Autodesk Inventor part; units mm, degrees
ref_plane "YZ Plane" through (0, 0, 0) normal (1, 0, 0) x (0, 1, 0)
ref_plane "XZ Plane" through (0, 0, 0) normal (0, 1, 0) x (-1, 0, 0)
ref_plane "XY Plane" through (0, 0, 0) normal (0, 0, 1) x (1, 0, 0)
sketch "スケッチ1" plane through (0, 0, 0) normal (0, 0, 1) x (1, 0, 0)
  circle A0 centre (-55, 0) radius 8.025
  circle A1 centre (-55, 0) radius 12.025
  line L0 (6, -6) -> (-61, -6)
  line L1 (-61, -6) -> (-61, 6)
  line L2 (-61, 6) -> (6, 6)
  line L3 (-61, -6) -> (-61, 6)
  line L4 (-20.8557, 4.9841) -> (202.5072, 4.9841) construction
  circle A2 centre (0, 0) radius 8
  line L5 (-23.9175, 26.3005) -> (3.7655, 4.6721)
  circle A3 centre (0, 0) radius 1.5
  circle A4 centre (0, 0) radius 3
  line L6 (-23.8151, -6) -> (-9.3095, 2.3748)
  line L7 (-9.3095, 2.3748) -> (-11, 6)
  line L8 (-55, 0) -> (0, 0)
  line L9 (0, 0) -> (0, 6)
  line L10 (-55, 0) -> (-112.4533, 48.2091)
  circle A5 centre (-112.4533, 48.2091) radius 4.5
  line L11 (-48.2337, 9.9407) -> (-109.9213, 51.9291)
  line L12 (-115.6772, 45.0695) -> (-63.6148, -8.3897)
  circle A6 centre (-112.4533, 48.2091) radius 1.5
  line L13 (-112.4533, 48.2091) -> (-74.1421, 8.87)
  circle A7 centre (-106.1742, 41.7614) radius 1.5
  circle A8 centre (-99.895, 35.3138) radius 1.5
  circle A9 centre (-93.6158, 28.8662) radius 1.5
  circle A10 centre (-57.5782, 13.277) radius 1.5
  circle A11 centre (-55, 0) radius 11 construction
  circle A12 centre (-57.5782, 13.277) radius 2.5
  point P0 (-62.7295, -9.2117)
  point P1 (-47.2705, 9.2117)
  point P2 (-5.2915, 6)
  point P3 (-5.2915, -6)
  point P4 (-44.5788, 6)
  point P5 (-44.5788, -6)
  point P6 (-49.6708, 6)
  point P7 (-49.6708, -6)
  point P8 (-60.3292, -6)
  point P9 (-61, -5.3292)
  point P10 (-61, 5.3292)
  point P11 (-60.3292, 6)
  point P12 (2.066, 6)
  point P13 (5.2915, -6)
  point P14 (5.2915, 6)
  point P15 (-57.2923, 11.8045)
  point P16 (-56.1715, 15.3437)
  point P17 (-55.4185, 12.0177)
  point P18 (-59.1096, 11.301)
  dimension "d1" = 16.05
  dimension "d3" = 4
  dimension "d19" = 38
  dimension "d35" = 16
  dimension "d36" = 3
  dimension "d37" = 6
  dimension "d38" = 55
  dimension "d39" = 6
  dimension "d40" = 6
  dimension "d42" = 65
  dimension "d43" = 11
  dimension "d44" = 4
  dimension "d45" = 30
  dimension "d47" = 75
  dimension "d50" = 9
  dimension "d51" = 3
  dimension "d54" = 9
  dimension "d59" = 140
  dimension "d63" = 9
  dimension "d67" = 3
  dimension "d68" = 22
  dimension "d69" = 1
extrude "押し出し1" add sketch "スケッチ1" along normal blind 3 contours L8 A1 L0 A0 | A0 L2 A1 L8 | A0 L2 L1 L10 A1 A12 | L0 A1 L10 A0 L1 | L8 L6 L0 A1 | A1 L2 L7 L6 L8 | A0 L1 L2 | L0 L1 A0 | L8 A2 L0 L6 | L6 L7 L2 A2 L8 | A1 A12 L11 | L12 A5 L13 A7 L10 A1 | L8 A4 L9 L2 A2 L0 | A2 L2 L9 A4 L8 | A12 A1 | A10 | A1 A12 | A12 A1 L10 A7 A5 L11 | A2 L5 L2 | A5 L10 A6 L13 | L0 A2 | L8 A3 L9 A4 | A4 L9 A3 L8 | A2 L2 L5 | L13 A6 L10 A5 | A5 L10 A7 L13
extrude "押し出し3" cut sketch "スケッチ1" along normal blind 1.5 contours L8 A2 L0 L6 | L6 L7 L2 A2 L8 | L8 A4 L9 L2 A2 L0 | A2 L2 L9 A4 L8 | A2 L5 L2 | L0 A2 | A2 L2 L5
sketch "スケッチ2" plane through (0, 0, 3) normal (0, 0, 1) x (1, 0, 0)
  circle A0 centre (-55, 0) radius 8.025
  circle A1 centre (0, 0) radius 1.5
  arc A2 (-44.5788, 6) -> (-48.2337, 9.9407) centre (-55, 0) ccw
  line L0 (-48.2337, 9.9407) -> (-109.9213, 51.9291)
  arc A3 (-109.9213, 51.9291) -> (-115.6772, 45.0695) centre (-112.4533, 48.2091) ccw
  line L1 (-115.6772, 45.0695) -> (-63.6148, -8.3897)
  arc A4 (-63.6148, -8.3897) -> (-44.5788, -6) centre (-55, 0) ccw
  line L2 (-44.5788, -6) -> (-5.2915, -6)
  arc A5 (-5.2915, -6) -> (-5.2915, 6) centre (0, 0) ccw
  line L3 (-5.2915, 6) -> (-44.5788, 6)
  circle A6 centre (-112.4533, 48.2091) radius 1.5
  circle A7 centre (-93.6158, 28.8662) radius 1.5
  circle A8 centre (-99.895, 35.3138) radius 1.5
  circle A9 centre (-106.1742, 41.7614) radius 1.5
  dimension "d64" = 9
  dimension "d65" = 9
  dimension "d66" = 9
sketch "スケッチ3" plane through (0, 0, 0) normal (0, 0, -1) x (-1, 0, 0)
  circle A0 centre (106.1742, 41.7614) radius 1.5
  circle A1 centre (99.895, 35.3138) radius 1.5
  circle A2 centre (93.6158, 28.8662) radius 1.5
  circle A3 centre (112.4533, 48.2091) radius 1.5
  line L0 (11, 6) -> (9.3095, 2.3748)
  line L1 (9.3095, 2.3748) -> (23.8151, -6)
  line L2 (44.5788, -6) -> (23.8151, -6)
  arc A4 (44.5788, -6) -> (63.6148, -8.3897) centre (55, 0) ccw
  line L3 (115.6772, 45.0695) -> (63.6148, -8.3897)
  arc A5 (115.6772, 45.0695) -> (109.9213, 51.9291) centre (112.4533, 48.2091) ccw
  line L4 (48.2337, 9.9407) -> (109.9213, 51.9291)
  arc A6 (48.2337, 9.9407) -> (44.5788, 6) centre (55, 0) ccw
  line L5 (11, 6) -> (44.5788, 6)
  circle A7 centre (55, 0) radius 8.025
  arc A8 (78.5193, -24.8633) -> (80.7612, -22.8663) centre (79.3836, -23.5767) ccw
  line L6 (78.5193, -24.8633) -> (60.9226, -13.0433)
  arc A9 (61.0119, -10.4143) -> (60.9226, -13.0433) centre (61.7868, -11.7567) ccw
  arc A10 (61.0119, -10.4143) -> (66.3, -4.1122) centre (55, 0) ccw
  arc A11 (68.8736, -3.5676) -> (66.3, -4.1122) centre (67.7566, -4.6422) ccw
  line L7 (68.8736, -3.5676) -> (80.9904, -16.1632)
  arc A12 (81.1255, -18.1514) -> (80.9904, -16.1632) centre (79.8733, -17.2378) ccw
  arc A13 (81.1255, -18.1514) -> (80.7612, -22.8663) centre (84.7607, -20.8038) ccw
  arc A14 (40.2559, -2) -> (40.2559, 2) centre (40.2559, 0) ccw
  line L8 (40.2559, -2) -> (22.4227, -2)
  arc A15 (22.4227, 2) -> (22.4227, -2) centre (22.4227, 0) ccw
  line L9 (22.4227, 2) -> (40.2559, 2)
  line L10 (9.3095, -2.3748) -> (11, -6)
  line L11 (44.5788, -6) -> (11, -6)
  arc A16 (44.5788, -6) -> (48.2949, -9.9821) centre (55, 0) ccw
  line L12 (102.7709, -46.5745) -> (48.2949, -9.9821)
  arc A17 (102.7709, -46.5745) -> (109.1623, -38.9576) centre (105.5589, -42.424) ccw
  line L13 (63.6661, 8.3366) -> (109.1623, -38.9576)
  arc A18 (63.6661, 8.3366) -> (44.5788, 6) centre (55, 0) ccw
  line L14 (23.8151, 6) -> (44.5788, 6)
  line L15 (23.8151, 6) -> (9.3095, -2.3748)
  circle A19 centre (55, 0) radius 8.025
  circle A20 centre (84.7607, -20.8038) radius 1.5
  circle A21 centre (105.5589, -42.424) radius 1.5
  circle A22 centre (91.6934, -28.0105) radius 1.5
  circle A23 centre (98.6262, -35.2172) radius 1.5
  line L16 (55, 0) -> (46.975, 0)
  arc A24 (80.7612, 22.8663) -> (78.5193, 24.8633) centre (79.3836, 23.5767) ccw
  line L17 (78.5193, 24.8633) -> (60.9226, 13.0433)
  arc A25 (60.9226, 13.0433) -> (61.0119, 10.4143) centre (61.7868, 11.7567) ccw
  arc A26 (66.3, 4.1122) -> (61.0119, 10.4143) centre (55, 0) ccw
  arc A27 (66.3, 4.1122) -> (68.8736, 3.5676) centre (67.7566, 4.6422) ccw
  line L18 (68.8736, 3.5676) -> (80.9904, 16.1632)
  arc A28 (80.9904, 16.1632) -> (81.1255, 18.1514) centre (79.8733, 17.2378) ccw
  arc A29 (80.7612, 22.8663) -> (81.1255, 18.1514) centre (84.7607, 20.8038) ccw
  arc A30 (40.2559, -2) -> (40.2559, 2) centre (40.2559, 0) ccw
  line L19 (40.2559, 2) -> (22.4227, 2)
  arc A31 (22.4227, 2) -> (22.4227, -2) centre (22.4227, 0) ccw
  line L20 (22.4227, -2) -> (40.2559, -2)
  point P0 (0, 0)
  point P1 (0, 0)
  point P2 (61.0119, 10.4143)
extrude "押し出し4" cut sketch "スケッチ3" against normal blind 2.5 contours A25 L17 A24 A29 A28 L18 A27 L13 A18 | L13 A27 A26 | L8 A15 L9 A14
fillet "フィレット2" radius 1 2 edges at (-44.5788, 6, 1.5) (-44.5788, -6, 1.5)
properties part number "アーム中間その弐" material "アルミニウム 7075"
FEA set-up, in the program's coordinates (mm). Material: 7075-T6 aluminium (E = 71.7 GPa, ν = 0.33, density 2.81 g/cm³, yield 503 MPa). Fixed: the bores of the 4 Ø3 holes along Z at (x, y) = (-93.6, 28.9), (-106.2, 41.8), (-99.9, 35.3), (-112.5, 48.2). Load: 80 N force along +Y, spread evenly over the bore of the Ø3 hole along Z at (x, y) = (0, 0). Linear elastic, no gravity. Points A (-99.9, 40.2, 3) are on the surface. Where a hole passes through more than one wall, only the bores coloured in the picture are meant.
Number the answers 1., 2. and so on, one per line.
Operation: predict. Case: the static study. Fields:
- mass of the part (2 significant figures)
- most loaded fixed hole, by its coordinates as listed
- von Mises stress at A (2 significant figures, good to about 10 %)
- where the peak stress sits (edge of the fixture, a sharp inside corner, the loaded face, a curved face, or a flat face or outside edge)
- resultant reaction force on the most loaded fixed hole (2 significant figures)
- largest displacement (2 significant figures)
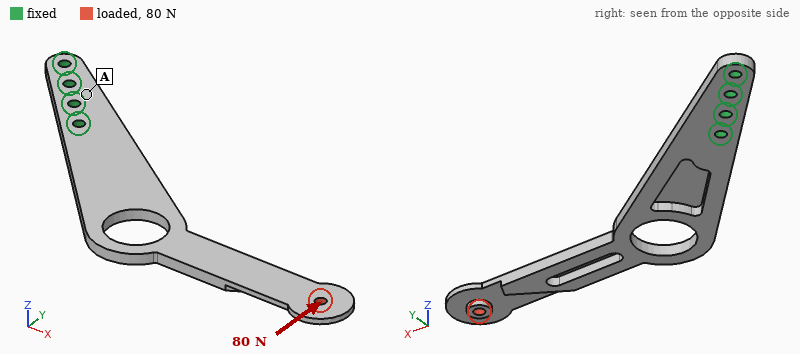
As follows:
1. 13 g
2. (-93.6, 28.9)
3. 15 MPa
4. a curved face
5. 590 N
6. 0.63 mm
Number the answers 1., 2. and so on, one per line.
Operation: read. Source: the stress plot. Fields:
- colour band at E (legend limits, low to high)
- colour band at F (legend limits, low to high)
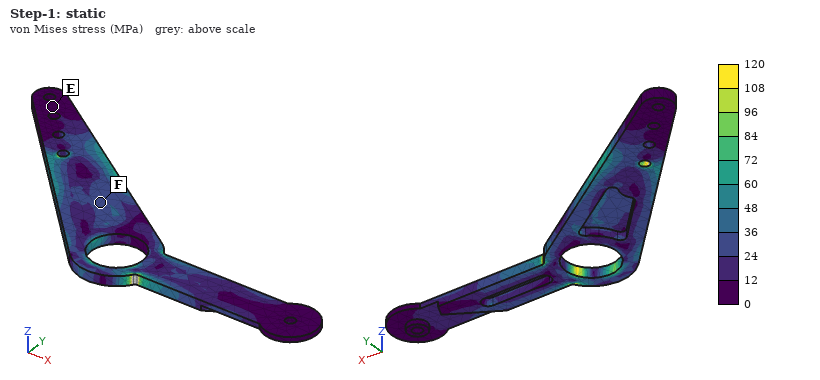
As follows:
1. 0 to 12 MPa
2. 24 to 36 MPa
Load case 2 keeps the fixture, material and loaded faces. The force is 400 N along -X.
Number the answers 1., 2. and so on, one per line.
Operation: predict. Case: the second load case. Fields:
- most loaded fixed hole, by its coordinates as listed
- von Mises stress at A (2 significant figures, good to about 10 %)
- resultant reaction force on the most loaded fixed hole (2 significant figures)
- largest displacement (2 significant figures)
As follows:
1. (-93.6, 28.9)
2. 22 MPa
3. 1.2 kN
4. 0.85 mm
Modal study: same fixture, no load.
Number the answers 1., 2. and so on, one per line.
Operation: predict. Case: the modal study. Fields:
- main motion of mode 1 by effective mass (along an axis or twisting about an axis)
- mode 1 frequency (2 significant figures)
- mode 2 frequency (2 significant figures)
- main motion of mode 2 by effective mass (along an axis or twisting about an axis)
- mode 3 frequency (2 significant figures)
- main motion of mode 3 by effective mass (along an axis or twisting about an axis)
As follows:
1. along Z
2. 260 Hz
3. 1100 Hz
4. along Z
5. 1300 Hz
6. along Y
